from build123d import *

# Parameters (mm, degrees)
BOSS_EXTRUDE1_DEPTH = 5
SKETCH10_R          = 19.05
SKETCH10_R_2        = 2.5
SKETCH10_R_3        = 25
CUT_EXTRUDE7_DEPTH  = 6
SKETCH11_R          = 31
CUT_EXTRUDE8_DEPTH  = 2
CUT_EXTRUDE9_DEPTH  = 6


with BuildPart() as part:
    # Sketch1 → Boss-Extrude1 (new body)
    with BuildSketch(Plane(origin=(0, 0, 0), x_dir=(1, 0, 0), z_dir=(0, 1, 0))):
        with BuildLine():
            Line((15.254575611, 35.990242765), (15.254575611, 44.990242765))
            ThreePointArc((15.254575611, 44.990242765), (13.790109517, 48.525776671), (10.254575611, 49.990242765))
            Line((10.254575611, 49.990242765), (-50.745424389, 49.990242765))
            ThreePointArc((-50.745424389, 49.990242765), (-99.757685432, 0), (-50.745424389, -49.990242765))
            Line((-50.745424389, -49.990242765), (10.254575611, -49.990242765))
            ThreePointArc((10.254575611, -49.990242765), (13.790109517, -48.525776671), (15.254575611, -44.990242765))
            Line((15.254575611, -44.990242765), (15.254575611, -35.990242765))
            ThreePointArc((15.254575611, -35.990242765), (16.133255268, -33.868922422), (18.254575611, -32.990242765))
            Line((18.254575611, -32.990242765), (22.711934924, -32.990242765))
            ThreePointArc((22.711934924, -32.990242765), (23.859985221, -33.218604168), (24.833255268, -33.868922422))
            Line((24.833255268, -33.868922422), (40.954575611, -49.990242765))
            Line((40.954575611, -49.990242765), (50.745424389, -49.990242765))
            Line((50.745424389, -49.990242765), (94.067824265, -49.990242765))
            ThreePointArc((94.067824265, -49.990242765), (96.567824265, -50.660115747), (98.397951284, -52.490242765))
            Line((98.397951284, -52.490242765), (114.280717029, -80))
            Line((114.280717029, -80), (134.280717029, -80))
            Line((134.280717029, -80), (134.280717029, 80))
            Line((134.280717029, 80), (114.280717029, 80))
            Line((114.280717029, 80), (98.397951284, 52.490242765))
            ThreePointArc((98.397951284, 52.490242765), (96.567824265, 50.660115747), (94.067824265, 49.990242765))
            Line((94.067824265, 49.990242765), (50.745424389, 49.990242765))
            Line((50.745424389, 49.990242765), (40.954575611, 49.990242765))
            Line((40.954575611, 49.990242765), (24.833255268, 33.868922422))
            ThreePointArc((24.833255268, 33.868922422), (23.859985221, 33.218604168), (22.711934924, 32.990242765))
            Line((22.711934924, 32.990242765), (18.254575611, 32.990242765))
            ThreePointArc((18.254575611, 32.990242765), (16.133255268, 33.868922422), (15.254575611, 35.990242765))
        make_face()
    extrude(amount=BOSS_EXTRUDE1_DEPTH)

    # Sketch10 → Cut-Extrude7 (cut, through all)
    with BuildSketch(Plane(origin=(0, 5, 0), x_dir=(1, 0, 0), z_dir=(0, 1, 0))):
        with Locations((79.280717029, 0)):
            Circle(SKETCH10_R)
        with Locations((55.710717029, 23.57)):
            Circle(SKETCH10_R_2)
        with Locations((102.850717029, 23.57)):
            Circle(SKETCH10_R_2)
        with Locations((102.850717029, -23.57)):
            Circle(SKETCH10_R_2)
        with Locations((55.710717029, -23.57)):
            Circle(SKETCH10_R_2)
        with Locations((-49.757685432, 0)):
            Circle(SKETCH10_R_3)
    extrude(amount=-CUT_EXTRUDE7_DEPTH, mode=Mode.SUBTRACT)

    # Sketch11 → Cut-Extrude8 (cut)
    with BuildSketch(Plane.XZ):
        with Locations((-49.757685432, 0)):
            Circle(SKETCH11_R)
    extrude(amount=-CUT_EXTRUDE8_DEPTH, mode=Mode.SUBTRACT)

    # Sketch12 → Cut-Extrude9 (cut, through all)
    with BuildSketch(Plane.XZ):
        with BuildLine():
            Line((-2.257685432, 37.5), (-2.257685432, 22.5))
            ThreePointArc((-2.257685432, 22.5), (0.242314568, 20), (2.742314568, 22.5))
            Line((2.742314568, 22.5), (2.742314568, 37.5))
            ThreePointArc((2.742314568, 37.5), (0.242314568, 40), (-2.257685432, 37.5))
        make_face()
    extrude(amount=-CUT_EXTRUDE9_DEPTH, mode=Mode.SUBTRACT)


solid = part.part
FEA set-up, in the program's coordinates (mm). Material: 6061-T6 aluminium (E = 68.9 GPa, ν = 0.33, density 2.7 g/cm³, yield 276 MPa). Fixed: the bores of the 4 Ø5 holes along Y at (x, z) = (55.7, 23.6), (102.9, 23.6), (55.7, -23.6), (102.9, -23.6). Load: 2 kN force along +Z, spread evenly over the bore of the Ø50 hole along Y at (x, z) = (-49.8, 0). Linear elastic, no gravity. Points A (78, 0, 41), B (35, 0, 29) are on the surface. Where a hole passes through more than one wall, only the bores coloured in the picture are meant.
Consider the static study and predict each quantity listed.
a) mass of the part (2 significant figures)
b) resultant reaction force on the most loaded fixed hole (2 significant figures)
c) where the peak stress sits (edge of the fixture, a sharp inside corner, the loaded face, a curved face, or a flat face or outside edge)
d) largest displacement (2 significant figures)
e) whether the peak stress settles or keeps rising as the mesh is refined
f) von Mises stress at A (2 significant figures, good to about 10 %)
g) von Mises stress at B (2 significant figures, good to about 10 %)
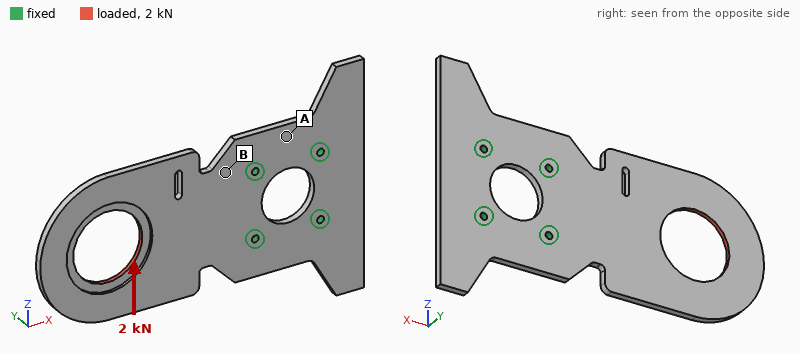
270 g
3.1 kN
edge of the fixture
0.19 mm
keeps rising
9.1 MPa
29 MPa
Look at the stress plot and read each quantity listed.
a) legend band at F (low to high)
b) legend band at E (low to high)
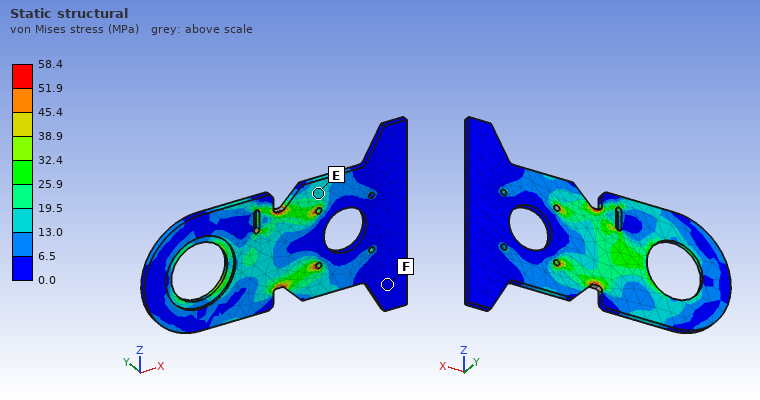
0.0 to 6.5 MPa
13.0 to 19.5 MPa
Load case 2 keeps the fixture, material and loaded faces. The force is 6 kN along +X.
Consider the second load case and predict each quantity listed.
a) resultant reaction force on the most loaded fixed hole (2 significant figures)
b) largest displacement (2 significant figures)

2.7 kN
1.2 mm
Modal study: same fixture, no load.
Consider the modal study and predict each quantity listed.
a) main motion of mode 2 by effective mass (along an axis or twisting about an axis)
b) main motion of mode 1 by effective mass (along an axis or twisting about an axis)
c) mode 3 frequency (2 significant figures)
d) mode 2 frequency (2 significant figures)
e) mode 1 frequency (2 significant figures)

twisting about X
along Y
950 Hz
580 Hz
190 Hz
